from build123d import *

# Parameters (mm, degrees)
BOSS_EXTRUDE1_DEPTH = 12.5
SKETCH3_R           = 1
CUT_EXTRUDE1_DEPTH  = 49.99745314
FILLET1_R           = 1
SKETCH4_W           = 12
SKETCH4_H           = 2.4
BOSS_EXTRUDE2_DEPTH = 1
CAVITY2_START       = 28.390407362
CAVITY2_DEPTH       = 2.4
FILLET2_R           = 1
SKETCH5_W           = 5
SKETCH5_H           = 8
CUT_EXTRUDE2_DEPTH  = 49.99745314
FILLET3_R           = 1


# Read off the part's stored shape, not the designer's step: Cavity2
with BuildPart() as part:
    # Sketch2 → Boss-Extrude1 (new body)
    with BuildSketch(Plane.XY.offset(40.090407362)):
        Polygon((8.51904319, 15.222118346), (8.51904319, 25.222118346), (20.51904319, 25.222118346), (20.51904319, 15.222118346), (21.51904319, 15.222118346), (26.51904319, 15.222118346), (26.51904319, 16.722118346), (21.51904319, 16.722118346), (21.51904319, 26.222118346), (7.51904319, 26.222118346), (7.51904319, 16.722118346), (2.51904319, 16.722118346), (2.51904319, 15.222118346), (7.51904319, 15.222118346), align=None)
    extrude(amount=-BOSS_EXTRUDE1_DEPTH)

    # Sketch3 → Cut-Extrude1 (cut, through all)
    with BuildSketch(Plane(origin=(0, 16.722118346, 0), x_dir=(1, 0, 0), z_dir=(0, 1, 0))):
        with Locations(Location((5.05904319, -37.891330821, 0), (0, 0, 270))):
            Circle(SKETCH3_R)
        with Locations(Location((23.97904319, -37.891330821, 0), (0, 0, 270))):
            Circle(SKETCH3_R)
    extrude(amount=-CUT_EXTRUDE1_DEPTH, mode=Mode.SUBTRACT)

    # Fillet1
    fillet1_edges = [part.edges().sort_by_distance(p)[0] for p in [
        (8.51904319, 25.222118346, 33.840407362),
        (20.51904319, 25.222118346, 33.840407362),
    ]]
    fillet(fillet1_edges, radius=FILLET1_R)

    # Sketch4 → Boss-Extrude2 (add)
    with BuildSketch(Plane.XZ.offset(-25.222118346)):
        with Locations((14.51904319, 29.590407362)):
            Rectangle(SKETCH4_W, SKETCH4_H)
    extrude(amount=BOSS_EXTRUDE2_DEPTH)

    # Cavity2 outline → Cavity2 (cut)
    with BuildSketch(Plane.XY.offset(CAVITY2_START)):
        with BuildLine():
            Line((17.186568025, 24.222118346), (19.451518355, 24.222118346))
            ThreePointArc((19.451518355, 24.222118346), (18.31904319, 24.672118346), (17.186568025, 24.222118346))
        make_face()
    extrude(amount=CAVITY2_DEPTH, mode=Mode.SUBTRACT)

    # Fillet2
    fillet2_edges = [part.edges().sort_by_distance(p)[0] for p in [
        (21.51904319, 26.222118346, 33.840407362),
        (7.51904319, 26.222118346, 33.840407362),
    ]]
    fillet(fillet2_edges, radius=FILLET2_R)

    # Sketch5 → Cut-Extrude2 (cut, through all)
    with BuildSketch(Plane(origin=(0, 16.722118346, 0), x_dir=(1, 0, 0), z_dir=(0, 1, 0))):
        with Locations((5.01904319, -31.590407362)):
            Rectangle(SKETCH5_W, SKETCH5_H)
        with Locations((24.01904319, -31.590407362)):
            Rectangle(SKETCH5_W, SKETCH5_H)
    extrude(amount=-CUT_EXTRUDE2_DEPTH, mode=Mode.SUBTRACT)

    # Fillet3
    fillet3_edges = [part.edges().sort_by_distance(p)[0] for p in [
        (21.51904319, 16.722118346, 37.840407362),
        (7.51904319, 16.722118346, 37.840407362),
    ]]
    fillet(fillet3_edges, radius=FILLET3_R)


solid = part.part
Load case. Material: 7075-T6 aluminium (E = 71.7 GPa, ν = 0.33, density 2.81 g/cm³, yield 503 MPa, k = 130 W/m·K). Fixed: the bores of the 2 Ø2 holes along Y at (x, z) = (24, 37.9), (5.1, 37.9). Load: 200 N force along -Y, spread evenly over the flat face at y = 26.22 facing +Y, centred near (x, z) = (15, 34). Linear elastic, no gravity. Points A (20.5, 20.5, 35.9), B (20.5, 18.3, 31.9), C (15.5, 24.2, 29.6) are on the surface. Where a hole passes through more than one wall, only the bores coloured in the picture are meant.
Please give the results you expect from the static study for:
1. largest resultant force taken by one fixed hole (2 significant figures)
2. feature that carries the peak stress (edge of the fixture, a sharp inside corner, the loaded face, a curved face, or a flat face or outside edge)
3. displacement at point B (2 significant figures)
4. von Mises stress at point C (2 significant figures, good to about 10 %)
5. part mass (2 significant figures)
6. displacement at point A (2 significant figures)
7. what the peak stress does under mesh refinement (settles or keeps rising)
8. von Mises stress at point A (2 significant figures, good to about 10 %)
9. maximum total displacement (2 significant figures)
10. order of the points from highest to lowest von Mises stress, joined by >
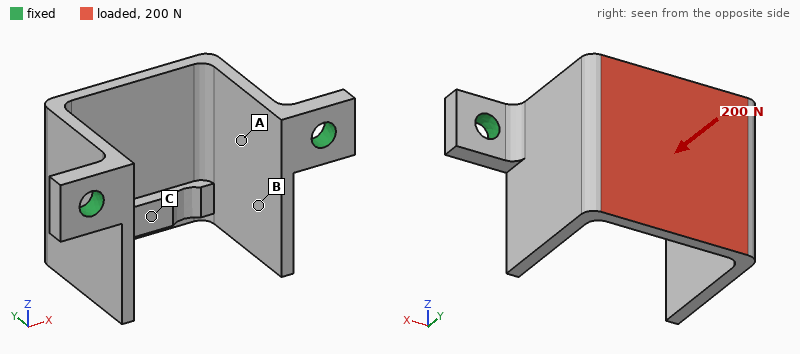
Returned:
100 N
edge of the fixture
0.042 mm
59 MPa
1.4 g
0.030 mm
keeps rising
37 MPa
0.10 mm
C > A > B
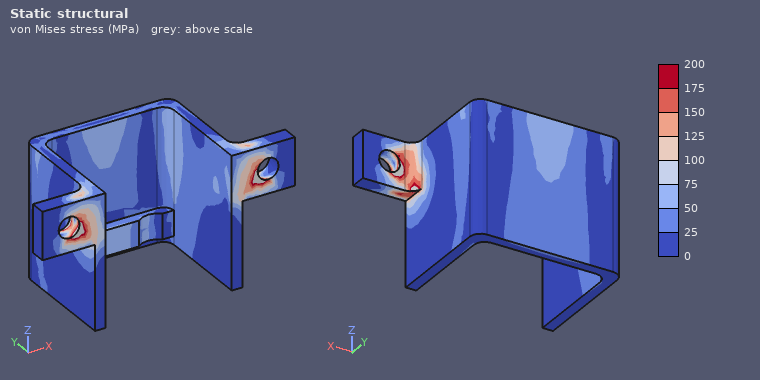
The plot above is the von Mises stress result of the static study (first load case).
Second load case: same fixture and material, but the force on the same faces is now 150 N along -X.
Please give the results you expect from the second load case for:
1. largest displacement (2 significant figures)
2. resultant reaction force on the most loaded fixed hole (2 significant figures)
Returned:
0.12 mm
100 N
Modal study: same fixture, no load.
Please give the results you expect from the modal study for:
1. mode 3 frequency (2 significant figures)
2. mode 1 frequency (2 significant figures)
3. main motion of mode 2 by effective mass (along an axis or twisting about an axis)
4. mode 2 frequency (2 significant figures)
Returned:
8600 Hz
5400 Hz
along X
5900 Hz
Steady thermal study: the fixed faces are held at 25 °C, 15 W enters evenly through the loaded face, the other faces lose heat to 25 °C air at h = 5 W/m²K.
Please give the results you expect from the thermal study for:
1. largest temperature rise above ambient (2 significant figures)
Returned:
87 K
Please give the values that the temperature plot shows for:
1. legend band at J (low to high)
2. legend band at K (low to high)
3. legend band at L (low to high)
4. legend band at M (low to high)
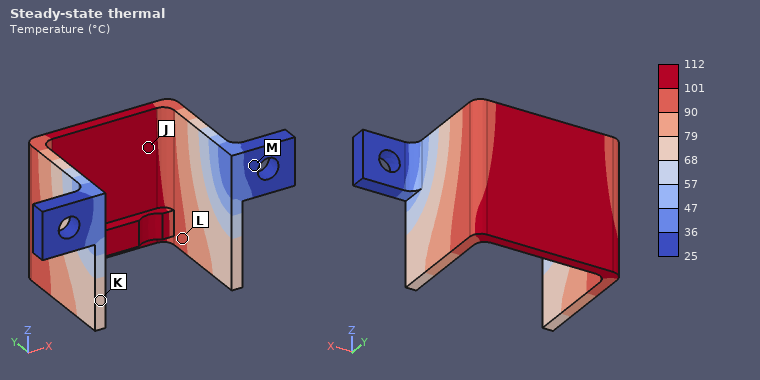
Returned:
101 to 112 °C
68 to 79 °C
90 to 101 °C
25 to 36 °C
